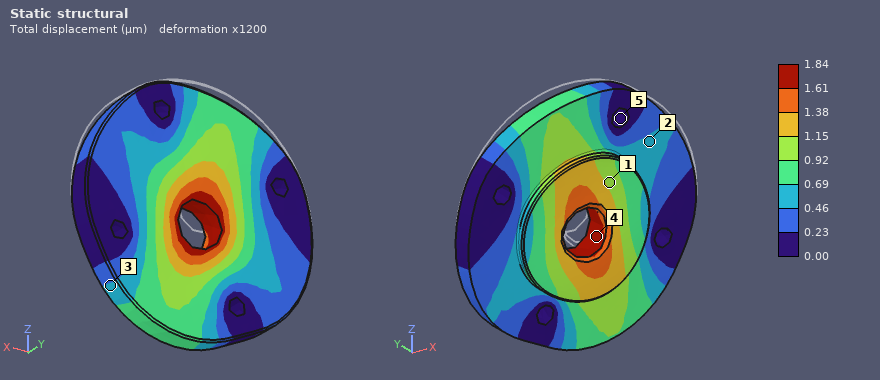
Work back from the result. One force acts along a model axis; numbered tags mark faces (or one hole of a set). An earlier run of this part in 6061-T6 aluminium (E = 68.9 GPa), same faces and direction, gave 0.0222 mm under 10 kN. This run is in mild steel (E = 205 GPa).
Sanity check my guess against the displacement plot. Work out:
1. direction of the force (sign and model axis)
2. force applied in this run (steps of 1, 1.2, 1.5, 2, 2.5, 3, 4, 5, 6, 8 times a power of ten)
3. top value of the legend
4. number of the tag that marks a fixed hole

-Z
2.5 kN
1.84 µm
5
